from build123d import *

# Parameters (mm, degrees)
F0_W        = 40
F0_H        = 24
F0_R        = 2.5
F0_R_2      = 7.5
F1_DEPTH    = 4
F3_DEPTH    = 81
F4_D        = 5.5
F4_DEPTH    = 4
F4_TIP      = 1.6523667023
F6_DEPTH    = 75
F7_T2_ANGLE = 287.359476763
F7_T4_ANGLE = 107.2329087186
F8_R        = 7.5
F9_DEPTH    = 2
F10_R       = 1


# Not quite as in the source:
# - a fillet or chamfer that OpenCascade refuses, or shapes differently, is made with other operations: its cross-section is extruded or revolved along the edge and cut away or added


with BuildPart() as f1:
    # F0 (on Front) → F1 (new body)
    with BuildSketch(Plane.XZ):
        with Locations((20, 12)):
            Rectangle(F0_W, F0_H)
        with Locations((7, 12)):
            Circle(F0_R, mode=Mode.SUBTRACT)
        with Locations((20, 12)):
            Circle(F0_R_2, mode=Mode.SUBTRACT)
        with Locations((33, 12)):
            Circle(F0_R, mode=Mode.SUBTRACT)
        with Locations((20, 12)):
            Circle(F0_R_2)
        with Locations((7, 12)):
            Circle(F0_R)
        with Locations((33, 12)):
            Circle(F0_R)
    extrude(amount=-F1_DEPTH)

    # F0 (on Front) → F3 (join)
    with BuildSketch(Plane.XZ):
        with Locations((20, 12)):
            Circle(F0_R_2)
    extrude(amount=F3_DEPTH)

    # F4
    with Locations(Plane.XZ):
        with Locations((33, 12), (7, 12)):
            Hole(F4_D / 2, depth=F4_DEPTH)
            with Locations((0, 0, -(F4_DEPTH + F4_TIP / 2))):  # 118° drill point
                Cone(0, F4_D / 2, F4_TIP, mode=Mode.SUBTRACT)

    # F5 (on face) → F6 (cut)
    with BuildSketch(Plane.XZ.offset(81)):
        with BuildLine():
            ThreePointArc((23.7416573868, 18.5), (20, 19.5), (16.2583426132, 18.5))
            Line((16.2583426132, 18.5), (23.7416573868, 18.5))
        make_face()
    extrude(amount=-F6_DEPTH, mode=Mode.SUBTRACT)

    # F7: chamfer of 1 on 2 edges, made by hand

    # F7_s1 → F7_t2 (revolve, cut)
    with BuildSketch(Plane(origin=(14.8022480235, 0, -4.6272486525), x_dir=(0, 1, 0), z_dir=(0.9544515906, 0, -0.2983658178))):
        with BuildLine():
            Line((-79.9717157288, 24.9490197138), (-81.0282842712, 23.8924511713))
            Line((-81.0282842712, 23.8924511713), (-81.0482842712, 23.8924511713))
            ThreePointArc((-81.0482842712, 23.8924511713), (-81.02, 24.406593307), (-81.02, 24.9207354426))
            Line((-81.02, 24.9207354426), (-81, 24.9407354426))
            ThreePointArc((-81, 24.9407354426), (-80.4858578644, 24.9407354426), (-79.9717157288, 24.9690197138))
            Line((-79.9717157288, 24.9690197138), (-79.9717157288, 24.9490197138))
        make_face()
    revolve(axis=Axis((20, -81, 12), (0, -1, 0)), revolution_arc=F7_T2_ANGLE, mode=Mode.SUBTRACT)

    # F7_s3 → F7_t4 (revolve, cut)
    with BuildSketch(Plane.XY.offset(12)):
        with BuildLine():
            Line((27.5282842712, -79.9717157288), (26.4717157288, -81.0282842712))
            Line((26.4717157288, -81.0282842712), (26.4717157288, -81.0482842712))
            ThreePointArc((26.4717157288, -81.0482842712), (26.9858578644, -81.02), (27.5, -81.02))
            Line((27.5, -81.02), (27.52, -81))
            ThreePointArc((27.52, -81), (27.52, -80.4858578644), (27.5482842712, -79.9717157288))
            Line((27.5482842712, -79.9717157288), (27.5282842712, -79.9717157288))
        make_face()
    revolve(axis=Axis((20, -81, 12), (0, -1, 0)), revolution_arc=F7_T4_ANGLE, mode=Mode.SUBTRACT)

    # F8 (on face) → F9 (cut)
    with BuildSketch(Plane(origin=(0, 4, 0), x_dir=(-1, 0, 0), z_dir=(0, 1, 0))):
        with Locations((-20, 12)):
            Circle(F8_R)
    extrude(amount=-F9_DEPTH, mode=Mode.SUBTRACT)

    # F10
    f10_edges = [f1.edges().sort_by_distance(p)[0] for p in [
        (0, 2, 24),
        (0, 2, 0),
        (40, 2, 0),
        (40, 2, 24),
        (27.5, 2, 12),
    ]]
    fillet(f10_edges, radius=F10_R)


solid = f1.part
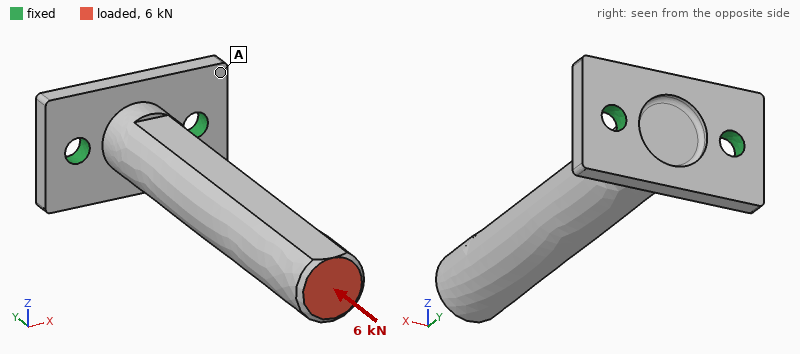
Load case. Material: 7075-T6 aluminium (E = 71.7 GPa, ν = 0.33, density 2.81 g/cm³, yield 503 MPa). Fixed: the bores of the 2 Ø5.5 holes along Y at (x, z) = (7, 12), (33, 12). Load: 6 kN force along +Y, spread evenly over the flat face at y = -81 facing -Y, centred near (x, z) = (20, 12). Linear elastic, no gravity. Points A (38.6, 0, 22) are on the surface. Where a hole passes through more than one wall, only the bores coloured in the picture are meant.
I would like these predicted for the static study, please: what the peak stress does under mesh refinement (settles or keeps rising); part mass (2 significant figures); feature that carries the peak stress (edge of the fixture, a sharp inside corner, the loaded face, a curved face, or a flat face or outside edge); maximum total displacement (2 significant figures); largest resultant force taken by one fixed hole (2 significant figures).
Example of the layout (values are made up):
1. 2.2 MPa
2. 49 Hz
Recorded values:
1. keeps rising
2. 48 g
3. edge of the fixture
4. 76 µm
5. 3.4 kN
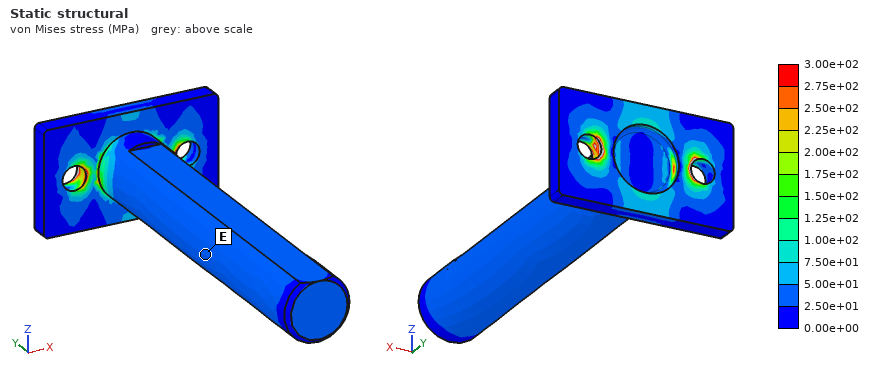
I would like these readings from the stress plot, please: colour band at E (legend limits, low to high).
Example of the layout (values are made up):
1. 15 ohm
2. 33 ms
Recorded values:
1. 2.50e+01 to 5.00e+01 MPa
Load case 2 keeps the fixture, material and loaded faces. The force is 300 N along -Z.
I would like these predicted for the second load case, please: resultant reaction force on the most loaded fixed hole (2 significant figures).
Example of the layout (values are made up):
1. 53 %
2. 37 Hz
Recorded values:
1. 150 N
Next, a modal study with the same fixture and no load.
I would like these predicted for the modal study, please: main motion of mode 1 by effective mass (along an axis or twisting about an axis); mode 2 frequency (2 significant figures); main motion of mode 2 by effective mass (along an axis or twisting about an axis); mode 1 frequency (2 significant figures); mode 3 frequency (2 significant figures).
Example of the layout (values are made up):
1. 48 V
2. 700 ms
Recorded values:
1. along Z
2. 1300 Hz
3. along X
4. 830 Hz
5. 6600 Hz
